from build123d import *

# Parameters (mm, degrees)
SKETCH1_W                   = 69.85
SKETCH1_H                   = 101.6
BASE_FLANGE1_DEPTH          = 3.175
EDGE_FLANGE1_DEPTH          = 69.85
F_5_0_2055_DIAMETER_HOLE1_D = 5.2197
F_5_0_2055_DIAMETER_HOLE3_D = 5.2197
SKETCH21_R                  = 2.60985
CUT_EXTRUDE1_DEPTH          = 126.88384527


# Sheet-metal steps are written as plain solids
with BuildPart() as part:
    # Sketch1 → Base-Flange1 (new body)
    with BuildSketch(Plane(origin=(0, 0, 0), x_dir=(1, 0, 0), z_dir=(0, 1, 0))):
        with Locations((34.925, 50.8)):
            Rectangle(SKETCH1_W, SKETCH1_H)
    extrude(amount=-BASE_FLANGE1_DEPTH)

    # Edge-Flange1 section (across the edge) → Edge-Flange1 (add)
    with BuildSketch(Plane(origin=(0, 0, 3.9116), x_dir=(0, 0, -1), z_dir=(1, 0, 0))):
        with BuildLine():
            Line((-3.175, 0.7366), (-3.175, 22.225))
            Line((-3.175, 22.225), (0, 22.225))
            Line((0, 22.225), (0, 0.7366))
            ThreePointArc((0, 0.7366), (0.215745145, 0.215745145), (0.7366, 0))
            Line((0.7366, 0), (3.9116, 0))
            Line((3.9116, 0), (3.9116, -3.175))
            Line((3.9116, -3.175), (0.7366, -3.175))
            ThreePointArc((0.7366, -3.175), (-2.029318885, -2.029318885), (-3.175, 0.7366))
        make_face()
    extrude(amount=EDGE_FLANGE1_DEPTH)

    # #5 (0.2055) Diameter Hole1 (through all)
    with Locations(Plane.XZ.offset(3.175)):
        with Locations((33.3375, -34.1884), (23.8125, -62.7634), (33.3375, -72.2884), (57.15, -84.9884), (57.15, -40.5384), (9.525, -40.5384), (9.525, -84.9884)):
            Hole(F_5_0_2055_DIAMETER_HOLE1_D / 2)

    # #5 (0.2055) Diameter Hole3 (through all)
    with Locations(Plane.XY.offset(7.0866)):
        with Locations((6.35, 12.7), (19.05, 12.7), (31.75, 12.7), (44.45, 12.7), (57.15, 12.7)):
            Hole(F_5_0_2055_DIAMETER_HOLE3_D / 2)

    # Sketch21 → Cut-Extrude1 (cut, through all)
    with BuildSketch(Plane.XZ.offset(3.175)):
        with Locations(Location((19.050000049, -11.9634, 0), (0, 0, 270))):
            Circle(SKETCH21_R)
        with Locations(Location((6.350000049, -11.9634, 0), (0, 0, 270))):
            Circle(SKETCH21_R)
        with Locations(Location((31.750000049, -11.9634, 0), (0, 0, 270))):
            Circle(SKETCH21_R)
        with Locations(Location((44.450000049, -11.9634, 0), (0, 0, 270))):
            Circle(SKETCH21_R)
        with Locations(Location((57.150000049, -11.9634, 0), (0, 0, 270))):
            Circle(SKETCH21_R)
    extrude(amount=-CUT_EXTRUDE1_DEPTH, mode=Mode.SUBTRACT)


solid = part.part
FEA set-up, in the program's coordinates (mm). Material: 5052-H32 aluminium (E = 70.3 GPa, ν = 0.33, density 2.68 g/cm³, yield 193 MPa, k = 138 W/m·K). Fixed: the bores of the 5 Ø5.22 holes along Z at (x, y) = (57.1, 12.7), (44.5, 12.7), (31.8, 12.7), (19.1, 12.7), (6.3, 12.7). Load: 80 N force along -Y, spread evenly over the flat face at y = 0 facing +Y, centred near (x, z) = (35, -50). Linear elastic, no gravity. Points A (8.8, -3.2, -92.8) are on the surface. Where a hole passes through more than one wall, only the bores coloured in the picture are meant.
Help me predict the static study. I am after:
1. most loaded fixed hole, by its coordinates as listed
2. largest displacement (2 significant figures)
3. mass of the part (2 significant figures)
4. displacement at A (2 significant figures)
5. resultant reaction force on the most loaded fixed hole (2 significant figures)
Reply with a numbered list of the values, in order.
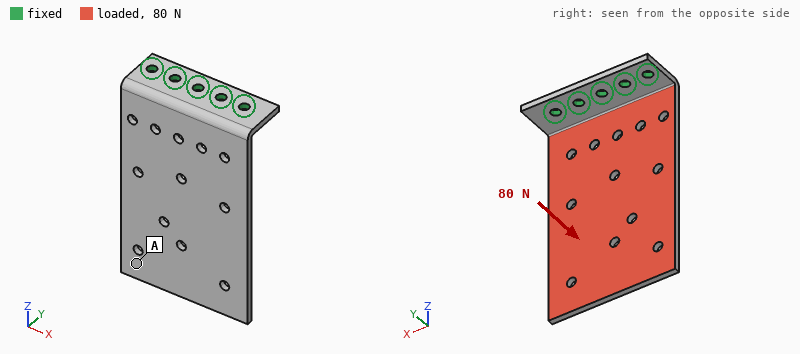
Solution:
1. (19.1, 12.7)
2. 1.4 mm
3. 74 g
4. 1.3 mm
5. 28 N
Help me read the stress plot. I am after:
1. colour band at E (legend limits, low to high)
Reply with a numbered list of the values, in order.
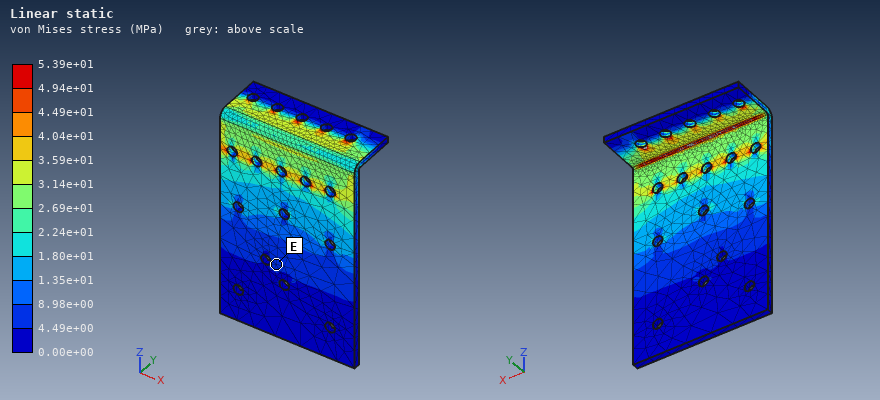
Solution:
1. 4.49e+00 to 8.98e+00 MPa
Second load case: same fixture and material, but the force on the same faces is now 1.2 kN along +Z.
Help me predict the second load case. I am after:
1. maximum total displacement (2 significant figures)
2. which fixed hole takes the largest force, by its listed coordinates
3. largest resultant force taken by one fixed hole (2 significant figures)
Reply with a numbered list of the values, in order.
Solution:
1. 0.14 mm
2. (57.1, 12.7)
3. 310 N
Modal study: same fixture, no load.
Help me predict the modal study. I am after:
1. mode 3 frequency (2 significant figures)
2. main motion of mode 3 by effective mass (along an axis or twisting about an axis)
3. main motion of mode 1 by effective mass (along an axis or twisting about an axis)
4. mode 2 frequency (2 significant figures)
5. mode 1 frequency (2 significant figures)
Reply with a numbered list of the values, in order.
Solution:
1. 1100 Hz
2. along X
3. along Y
4. 700 Hz
5. 190 Hz
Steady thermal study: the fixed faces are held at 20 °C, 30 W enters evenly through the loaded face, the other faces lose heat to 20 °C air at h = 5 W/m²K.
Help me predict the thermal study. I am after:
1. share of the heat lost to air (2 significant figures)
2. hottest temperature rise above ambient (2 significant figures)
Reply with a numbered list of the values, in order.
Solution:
1. 7.1 %
2. 65 K
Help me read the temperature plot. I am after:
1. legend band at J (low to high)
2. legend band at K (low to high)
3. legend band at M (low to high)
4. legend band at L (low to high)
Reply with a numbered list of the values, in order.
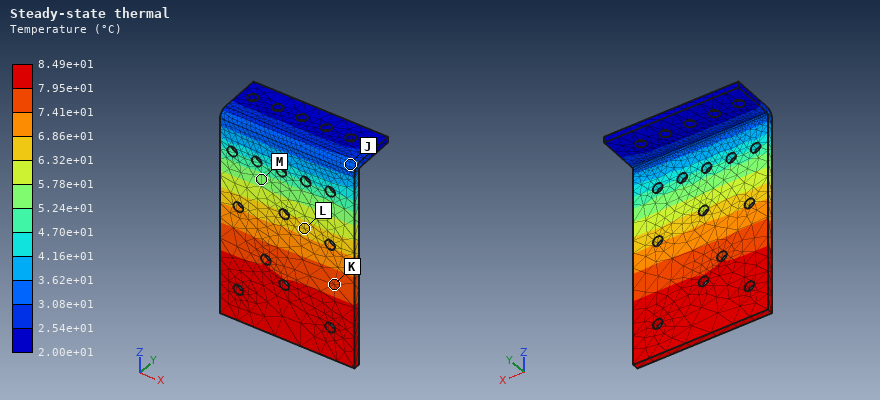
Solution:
1. 3.08e+01 to 3.62e+01 °C
2. 7.41e+01 to 7.95e+01 °C
3. 5.24e+01 to 5.78e+01 °C
4. 6.32e+01 to 6.86e+01 °C
